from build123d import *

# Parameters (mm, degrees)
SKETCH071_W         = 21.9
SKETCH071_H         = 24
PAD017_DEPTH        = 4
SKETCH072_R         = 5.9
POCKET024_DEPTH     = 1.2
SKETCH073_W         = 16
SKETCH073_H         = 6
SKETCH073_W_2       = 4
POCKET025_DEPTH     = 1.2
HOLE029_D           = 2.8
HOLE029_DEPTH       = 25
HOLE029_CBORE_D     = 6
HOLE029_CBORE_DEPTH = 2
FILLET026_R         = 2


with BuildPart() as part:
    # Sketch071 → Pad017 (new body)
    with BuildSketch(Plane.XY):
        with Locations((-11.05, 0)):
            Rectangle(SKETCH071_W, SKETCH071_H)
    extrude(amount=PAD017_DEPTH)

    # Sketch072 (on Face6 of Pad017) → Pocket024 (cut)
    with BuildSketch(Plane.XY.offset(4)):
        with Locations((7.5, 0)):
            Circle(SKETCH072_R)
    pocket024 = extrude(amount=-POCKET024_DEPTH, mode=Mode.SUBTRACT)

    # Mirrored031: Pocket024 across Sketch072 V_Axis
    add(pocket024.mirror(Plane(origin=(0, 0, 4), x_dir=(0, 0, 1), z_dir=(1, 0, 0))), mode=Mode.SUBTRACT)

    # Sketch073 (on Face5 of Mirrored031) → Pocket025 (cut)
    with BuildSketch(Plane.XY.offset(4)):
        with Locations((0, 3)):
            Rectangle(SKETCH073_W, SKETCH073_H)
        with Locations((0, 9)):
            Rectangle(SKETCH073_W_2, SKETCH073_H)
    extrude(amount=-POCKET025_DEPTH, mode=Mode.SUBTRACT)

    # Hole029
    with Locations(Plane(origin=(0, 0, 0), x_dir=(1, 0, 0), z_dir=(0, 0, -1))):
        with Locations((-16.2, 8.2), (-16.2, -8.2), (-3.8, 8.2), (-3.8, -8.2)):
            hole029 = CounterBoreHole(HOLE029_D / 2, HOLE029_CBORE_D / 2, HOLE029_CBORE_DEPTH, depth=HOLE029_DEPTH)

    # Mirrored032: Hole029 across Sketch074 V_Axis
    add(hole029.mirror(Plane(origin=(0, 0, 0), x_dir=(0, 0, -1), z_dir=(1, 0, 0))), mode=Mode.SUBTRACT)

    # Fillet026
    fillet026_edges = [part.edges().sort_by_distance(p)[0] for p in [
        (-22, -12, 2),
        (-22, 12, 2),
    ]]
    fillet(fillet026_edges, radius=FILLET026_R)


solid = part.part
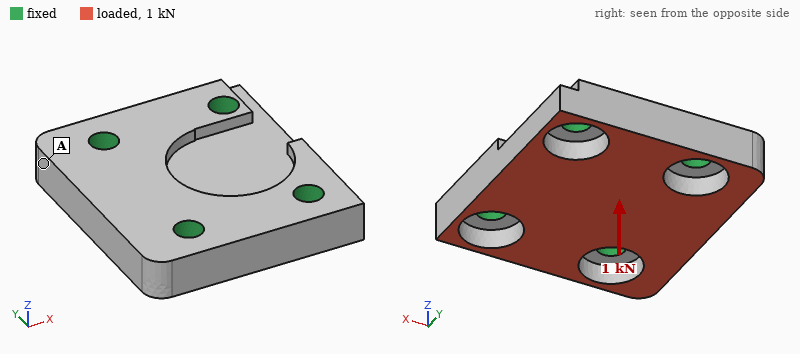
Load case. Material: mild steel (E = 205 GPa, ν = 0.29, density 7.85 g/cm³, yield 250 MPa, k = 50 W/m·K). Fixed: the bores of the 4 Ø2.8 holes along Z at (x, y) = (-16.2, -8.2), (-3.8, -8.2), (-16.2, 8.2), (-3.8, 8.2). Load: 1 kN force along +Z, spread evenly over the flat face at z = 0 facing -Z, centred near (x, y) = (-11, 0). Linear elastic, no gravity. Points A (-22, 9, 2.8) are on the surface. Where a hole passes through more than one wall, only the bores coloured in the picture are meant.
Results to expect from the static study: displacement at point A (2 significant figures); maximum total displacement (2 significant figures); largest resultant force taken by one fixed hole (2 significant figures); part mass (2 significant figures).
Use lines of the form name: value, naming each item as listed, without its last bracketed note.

displacement at point A: 0.89 µm
maximum total displacement: 1.8 µm
largest resultant force taken by one fixed hole: 310 N
part mass: 13 g
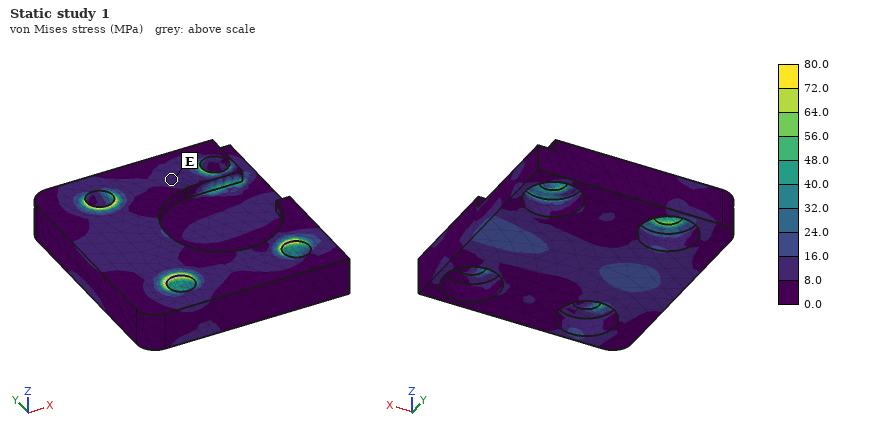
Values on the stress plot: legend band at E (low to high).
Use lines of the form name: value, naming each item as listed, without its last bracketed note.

legend band at E: 8.0 to 16.0 MPa
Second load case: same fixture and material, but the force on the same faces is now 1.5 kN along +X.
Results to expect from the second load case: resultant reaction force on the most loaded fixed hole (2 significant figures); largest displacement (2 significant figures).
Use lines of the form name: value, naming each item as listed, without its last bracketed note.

resultant reaction force on the most loaded fixed hole: 440 N
largest displacement: 2.9 µm
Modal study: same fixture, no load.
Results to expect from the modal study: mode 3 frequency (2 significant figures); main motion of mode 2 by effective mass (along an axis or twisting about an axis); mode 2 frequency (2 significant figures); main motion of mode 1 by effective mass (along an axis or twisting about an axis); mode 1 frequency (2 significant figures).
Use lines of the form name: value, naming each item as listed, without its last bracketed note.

mode 3 frequency: 55 kHz
main motion of mode 2 by effective mass: along Z
mode 2 frequency: 45 kHz
main motion of mode 1 by effective mass: along Z
mode 1 frequency: 39 kHz
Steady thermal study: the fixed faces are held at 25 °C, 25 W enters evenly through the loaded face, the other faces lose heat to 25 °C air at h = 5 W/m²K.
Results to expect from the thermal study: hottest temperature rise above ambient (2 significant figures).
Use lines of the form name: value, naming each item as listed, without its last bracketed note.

hottest temperature rise above ambient: 23 K
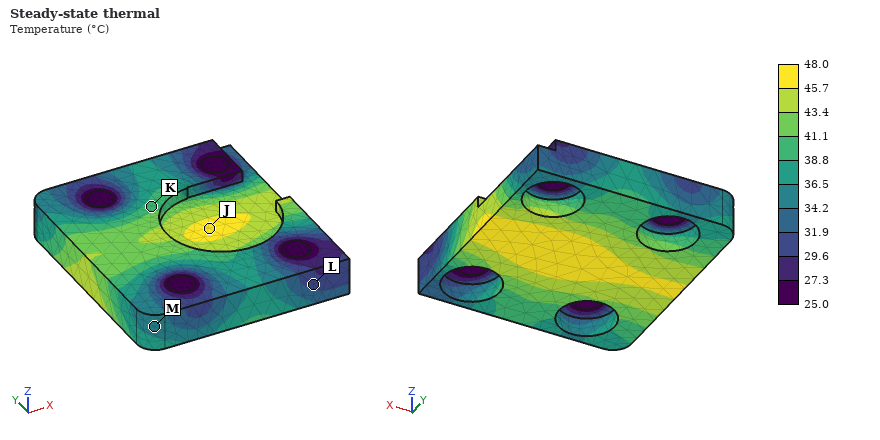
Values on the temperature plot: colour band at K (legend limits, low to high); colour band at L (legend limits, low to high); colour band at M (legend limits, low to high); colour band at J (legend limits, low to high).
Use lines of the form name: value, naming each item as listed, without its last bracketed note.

colour band at K: 38.8 to 41.1 °C
colour band at L: 29.6 to 31.9 °C
colour band at M: 34.2 to 36.5 °C
colour band at J: 45.7 to 48.0 °C
